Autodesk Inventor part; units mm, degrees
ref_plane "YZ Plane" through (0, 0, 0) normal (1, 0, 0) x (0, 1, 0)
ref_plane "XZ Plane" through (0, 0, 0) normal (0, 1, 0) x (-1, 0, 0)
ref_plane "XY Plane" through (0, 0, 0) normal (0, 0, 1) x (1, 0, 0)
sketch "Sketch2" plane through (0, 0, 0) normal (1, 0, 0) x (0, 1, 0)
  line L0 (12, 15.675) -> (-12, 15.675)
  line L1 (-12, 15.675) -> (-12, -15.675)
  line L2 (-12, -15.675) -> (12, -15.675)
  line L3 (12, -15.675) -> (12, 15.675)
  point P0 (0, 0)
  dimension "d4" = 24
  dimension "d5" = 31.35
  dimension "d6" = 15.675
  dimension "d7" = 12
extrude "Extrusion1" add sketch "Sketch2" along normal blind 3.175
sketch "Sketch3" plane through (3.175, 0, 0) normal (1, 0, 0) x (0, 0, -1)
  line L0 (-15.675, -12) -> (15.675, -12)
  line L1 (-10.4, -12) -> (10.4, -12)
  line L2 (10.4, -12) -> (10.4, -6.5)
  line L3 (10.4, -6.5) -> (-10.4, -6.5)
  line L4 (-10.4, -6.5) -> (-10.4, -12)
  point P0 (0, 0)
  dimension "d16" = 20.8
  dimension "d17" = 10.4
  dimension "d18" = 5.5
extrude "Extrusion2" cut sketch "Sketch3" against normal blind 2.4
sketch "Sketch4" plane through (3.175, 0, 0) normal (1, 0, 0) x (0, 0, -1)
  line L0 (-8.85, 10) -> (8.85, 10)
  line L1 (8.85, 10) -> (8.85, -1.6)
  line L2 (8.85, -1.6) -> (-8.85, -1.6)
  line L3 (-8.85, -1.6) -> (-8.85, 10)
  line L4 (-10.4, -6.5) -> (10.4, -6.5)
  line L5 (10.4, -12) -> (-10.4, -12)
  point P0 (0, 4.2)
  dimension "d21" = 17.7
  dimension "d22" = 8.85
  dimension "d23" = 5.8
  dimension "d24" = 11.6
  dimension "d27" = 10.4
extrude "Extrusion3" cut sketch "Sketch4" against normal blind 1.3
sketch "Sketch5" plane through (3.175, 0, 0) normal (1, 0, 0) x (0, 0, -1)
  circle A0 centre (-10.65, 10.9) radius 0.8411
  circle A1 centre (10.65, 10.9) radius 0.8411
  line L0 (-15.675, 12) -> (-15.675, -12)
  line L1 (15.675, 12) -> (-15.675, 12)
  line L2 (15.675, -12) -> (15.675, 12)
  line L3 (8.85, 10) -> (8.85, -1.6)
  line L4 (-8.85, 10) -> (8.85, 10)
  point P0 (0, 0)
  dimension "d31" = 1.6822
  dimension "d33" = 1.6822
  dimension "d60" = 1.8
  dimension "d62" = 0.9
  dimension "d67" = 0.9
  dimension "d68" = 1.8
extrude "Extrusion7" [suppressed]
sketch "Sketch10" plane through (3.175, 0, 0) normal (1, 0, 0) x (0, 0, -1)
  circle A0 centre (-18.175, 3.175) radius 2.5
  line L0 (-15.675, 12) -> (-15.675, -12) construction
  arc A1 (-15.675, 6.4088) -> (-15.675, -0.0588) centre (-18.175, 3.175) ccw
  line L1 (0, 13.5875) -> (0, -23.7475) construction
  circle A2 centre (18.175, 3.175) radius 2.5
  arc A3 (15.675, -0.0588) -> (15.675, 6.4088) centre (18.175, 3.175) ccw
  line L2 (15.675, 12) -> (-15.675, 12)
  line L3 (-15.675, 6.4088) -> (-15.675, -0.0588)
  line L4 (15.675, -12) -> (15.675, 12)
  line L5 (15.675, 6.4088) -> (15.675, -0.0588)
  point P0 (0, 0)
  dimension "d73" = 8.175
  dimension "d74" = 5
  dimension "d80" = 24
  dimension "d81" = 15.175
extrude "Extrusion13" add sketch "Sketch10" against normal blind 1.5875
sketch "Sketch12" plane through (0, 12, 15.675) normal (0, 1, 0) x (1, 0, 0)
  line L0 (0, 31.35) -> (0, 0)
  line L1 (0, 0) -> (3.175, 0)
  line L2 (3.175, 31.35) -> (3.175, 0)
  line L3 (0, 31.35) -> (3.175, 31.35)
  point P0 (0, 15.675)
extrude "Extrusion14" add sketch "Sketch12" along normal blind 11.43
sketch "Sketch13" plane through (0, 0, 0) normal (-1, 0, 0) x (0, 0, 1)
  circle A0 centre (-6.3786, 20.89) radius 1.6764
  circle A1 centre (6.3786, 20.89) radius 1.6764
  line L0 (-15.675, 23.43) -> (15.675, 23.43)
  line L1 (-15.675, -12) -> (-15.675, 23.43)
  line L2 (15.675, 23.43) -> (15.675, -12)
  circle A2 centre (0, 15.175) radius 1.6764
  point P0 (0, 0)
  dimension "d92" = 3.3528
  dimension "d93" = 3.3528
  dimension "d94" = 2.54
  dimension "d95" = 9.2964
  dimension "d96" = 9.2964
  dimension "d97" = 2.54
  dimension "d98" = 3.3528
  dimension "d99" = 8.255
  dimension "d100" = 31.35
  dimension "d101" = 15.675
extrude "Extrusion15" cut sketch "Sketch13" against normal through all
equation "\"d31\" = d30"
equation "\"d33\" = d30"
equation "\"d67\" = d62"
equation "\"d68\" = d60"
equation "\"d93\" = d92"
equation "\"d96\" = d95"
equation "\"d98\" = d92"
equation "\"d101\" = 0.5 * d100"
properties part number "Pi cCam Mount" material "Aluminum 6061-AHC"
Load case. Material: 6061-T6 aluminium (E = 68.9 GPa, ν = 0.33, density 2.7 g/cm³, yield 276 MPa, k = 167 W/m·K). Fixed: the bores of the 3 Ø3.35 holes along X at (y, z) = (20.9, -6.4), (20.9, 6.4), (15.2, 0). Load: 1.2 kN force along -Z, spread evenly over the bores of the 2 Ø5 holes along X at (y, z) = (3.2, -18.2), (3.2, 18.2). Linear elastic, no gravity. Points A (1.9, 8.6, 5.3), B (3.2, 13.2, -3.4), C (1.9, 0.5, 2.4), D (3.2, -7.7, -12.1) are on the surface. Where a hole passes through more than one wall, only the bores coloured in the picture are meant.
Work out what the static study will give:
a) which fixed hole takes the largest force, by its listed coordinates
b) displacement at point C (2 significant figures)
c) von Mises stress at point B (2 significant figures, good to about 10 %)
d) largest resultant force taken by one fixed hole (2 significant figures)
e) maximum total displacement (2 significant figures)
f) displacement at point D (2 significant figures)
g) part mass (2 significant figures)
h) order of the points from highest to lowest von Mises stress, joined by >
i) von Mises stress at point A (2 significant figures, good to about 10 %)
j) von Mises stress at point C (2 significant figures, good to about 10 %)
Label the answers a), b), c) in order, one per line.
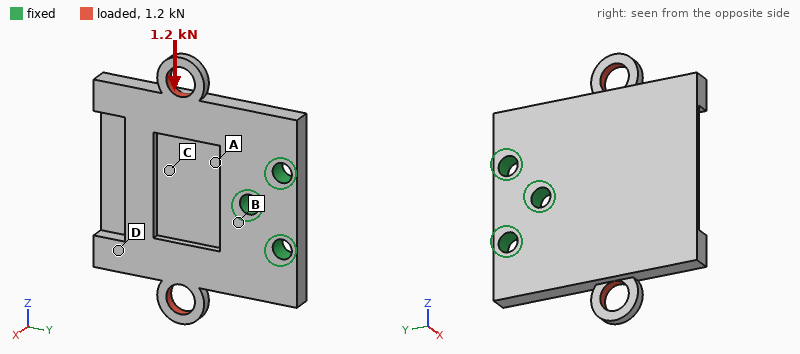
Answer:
a) (15.2, 0)
b) 22 µm
c) 69 MPa
d) 1.5 kN
e) 83 µm
f) 55 µm
g) 8.1 g
h) B > A > C > D
i) 56 MPa
j) 33 MPa
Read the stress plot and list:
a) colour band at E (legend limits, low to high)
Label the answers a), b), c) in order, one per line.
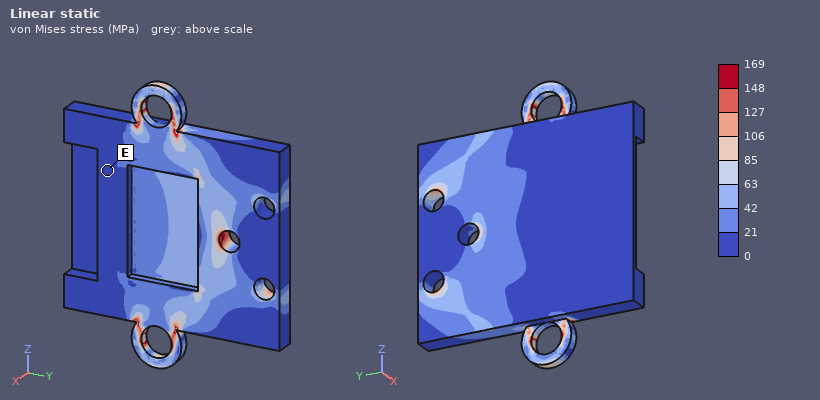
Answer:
a) 0 to 21 MPa
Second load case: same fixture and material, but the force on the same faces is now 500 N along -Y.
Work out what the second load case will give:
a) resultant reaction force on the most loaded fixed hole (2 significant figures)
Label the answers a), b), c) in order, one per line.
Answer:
a) 200 N
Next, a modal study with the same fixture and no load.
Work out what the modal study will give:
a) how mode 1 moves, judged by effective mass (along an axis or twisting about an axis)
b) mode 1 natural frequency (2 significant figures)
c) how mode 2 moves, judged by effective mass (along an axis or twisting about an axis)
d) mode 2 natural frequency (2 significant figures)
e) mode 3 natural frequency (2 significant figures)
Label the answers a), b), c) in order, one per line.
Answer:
a) along X
b) 3300 Hz
c) twisting about Y
d) 4700 Hz
e) 12 kHz
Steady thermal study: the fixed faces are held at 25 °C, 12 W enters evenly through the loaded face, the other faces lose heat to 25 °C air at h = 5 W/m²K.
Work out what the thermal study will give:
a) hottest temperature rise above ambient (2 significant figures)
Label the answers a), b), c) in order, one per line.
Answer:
a) 39 K
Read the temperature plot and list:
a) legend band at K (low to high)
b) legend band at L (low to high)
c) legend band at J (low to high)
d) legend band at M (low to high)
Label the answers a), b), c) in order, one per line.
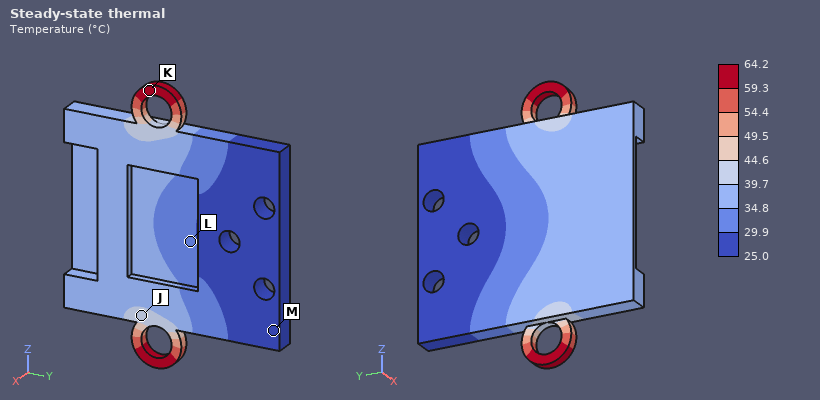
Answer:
a) 59.3 to 64.2 °C
b) 29.9 to 34.8 °C
c) 39.7 to 44.6 °C
d) 25.0 to 29.9 °C
